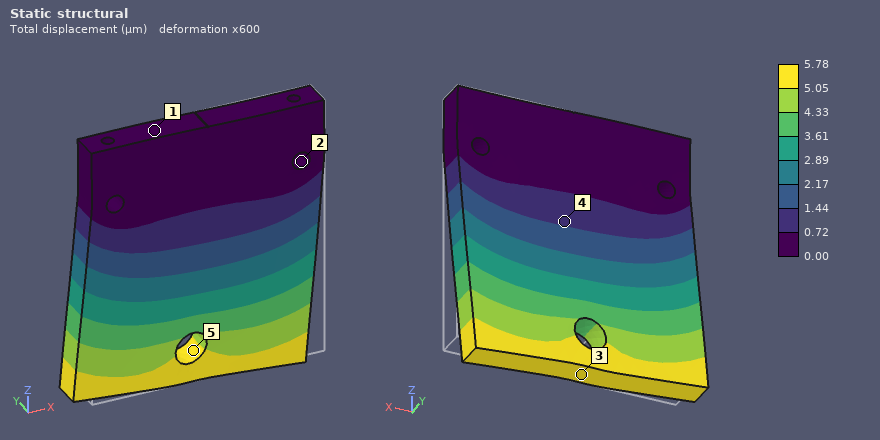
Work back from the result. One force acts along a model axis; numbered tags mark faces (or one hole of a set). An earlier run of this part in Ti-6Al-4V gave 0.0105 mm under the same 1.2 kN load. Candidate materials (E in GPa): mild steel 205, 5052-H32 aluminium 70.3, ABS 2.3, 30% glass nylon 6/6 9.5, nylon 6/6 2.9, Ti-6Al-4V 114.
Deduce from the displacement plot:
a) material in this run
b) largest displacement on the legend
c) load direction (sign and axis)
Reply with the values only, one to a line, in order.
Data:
mild steel
5.78 µm
-X
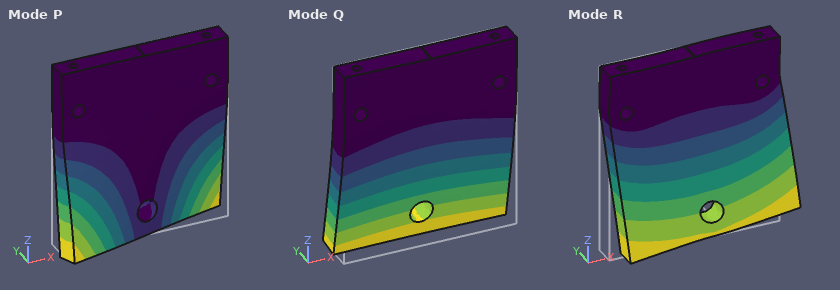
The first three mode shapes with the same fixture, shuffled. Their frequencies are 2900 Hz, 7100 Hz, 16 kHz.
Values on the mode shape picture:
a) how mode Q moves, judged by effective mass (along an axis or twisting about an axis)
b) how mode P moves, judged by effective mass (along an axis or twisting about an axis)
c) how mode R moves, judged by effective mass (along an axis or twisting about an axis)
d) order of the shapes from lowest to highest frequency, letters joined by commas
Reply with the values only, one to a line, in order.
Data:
along Y
twisting about Z
along X
Q, P, R
